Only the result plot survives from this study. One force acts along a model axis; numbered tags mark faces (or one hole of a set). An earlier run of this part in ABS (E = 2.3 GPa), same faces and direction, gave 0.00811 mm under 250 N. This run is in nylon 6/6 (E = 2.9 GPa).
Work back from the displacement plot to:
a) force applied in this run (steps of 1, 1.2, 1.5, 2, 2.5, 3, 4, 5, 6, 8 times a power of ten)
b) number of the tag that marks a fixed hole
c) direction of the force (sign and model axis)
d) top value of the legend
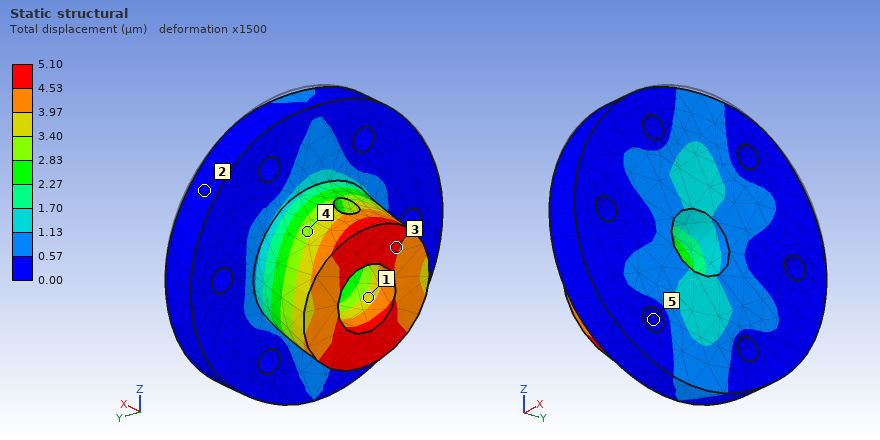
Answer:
200 N
5
-Z
5.10 µm
